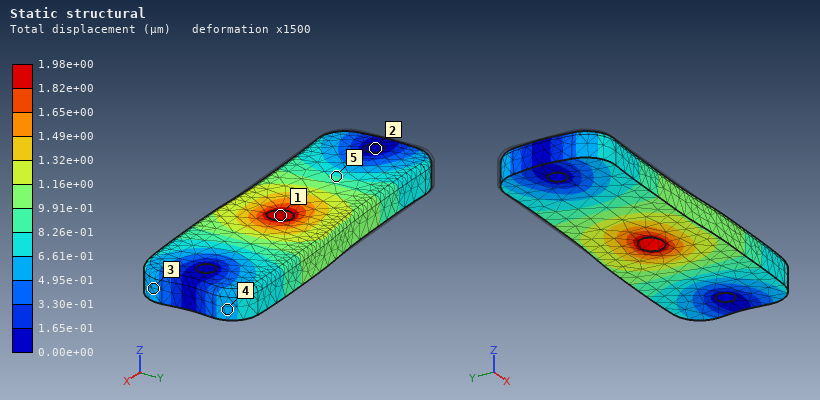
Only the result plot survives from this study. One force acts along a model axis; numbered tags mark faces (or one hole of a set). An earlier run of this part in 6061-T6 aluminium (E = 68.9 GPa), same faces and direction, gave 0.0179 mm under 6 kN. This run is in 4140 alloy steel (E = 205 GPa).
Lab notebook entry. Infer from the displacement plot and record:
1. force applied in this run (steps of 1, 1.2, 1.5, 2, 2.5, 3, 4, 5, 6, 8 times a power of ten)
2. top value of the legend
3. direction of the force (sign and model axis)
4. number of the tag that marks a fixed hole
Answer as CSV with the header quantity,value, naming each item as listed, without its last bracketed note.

quantity,value
force applied in this run,2 kN
top value of the legend,1.98e+00 µm
direction of the force,+X
number of the tag that marks a fixed hole,2
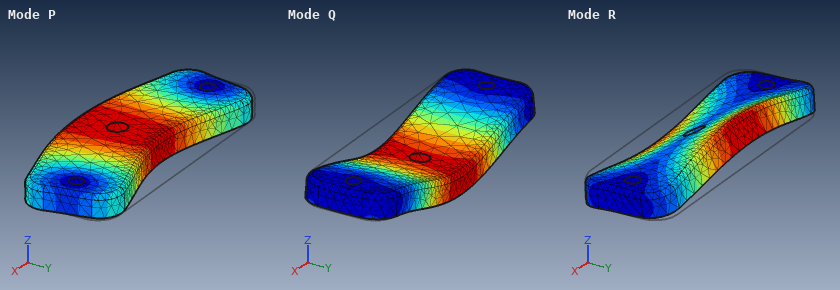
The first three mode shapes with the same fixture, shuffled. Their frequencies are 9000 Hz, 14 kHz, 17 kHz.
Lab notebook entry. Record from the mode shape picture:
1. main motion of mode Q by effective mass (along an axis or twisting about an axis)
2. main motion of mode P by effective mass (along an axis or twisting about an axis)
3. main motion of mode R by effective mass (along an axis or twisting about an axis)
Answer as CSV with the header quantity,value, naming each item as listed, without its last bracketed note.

quantity,value
main motion of mode Q by effective mass,along Z
main motion of mode P by effective mass,along Y
main motion of mode R by effective mass,twisting about X
